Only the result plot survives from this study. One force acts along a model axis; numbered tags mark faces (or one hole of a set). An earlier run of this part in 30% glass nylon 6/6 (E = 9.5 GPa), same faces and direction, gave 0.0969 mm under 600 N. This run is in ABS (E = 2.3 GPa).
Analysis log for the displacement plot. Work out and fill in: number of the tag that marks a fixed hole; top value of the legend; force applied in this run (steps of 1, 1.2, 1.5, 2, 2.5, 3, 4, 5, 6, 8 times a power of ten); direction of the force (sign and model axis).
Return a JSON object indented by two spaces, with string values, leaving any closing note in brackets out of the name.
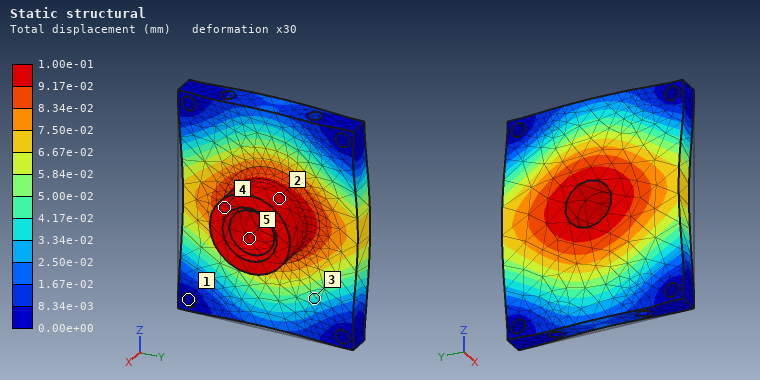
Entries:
{
  "number of the tag that marks a fixed hole": "1",
  "top value of the legend": "1.00e-01 mm",
  "force applied in this run": "150 N",
  "direction of the force": "-X"
}
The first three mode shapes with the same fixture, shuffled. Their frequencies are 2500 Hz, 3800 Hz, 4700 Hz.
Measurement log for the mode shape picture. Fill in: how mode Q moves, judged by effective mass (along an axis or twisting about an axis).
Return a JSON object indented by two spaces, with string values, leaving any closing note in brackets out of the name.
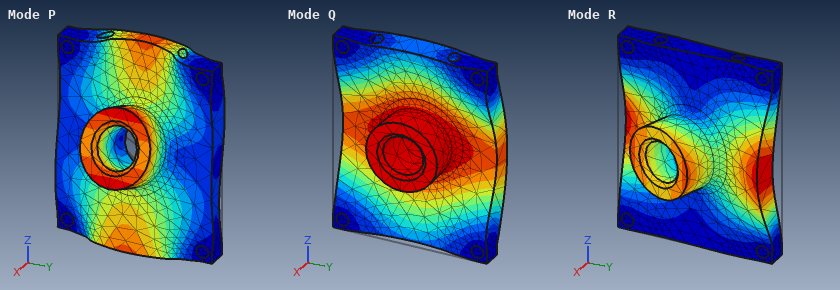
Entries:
{
  "how mode Q moves, judged by effective mass": "along X"
}
